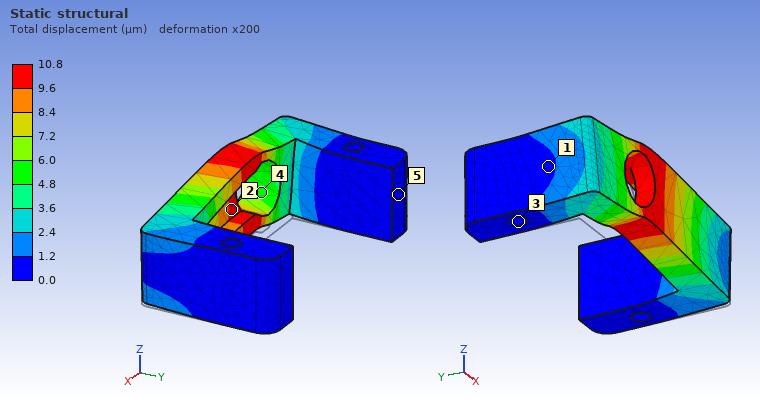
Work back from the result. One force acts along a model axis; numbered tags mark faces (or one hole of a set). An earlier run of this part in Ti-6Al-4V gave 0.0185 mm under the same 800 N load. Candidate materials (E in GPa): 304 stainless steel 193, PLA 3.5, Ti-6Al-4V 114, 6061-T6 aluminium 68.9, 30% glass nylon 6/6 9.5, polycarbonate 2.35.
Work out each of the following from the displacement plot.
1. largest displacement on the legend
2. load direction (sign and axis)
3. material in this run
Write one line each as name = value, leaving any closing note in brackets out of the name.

largest displacement on the legend = 10.8 µm
load direction = +Z
material in this run = 304 stainless steel
